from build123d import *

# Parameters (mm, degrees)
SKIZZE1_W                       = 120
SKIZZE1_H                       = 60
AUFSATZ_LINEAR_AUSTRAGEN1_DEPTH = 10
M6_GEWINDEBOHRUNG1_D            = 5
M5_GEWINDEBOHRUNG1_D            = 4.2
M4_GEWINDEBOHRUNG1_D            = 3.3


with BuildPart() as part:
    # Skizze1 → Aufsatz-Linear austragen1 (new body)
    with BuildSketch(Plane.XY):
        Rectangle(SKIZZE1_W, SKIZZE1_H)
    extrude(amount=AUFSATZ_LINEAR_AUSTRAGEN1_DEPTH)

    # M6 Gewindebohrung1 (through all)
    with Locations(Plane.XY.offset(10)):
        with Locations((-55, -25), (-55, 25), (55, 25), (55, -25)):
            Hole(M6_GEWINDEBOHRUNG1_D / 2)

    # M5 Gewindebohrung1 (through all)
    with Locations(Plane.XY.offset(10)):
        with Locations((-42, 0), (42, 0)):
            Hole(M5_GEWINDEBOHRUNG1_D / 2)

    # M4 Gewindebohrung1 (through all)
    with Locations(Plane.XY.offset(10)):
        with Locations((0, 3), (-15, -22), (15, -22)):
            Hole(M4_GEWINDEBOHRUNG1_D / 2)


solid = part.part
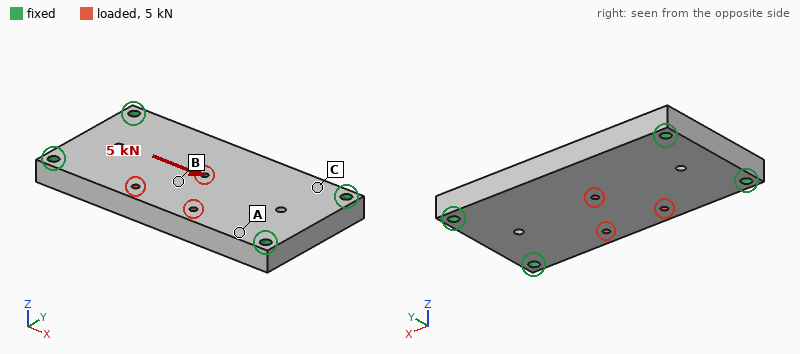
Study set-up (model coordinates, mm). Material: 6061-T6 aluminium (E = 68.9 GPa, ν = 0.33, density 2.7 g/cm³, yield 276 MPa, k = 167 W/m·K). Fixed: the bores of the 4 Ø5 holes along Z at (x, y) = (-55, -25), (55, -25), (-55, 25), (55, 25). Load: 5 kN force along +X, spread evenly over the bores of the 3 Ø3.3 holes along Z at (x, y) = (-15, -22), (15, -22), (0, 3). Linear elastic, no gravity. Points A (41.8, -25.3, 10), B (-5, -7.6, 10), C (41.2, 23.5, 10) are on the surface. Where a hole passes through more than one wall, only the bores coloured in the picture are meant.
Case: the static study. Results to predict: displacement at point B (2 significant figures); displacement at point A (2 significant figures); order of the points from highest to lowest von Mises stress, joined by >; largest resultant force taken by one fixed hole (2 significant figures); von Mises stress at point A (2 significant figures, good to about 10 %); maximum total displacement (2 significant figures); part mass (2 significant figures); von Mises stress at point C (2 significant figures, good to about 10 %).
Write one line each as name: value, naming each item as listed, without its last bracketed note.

displacement at point B: 4.2 µm
displacement at point A: 2.0 µm
order of the points from highest to lowest von Mises stress, joined by >: A > C > B
largest resultant force taken by one fixed hole: 1.5 kN
von Mises stress at point A: 9.7 MPa
maximum total displacement: 6.1 µm
part mass: 190 g
von Mises stress at point C: 5.3 MPa
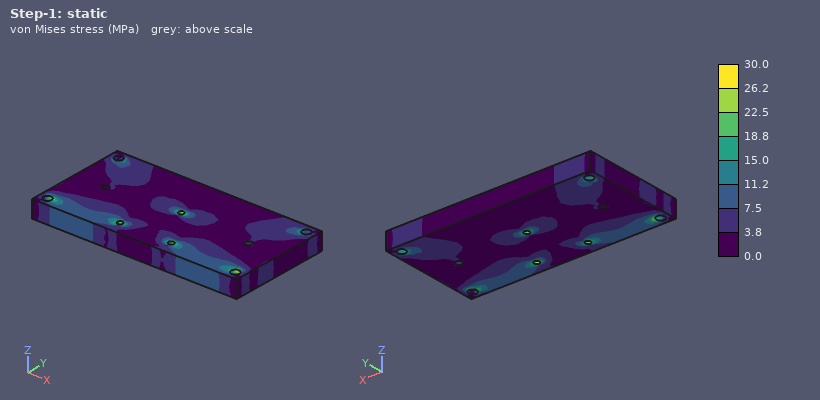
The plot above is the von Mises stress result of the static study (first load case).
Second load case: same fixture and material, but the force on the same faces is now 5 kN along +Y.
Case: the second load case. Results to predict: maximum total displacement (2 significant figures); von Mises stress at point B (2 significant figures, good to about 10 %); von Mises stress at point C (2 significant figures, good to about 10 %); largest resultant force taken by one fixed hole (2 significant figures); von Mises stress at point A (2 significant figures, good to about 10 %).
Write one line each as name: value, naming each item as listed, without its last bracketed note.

maximum total displacement: 13 µm
von Mises stress at point B: 3.6 MPa
von Mises stress at point C: 7.5 MPa
largest resultant force taken by one fixed hole: 1.8 kN
von Mises stress at point A: 6.5 MPa
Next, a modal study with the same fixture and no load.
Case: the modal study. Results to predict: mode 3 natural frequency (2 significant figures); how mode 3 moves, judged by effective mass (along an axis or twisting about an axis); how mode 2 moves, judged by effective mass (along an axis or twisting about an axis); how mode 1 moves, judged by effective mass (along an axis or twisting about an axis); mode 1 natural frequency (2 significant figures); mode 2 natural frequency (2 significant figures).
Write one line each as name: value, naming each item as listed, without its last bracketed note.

mode 3 natural frequency: 9300 Hz
how mode 3 moves, judged by effective mass: twisting about Y
how mode 2 moves, judged by effective mass: twisting about X
how mode 1 moves, judged by effective mass: along Z
mode 1 natural frequency: 3500 Hz
mode 2 natural frequency: 6000 Hz
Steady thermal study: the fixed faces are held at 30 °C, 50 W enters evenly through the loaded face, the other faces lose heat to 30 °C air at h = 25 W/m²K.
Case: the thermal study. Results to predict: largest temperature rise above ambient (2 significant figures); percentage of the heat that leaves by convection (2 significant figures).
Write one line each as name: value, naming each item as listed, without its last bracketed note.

largest temperature rise above ambient: 16 K
percentage of the heat that leaves by convection: 6.4 %
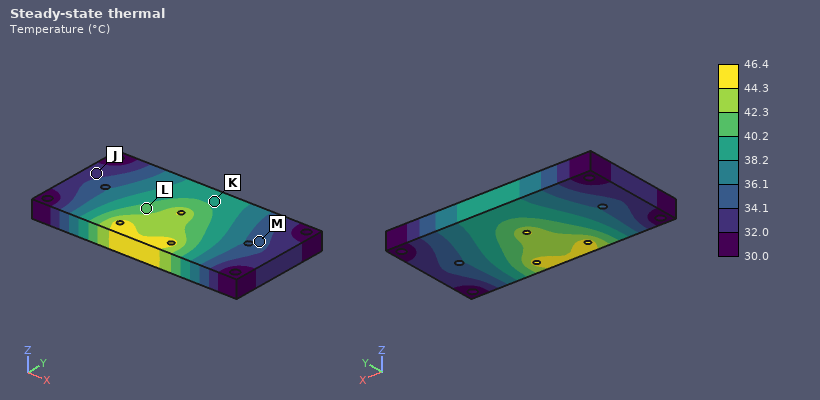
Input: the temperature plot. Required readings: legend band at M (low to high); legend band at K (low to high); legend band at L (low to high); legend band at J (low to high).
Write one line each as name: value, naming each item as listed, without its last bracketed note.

legend band at M: 34.1 to 36.1 °C
legend band at K: 38.2 to 40.2 °C
legend band at L: 40.2 to 42.3 °C
legend band at J: 32.0 to 34.1 °C
